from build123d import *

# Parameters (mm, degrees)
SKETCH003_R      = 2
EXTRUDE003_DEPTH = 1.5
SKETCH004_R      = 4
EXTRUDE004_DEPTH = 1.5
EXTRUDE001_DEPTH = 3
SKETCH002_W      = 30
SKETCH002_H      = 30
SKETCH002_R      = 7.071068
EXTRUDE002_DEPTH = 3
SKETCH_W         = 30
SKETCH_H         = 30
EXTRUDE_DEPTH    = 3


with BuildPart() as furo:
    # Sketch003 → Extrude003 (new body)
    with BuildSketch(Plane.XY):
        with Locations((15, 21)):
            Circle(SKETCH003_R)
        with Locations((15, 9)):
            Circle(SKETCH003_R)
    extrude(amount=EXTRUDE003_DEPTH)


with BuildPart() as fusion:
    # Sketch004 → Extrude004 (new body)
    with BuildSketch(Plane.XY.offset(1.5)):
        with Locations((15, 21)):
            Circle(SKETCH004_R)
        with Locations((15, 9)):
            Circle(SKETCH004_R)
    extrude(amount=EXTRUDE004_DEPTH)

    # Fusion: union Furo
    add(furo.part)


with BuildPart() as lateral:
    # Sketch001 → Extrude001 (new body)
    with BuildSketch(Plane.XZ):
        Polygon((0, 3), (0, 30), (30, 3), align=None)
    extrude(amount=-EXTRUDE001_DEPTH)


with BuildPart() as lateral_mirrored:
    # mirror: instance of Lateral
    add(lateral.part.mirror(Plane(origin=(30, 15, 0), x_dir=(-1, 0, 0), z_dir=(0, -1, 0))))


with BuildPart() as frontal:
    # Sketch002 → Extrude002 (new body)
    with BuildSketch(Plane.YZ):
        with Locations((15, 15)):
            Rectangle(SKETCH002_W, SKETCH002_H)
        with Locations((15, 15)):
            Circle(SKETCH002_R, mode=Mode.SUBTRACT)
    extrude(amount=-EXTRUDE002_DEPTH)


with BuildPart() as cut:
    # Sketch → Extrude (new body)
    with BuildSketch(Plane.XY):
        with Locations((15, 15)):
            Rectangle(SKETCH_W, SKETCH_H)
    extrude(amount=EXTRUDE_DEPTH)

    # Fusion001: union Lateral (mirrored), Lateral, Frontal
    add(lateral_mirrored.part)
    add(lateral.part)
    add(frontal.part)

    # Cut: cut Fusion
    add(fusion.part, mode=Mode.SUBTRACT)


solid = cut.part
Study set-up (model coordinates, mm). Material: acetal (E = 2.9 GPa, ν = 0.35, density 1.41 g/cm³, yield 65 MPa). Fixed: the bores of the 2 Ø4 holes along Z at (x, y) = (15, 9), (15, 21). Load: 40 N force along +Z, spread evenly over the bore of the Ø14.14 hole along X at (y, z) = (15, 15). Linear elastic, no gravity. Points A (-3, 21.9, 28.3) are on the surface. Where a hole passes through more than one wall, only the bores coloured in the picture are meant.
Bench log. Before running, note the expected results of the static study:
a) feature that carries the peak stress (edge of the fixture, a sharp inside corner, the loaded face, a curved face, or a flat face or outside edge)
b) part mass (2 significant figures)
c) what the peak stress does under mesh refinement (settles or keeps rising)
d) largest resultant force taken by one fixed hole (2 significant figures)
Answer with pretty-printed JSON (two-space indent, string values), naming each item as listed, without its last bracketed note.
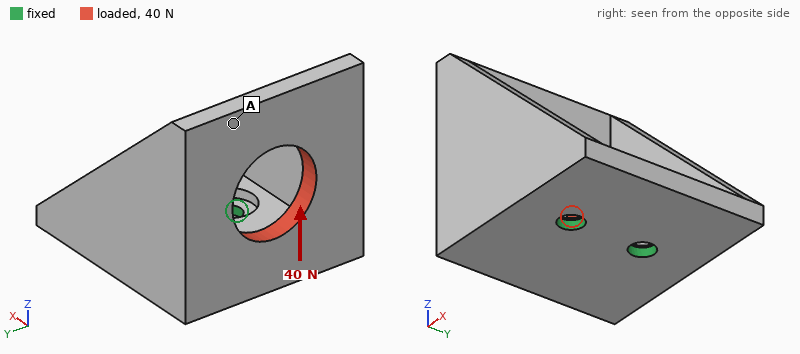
{
  "feature that carries the peak stress": "edge of the fixture",
  "part mass": "10 g",
  "what the peak stress does under mesh refinement": "keeps rising",
  "largest resultant force taken by one fixed hole": "21 N"
}
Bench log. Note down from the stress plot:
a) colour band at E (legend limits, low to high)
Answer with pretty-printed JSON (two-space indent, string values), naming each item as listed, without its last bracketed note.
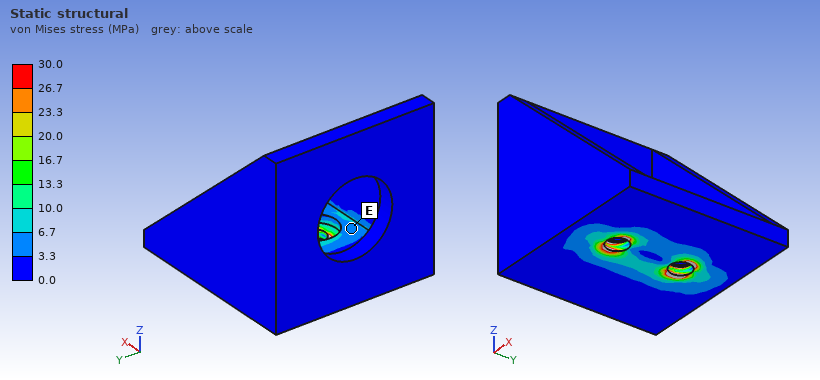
{
  "colour band at E": "3.3 to 6.7 MPa"
}
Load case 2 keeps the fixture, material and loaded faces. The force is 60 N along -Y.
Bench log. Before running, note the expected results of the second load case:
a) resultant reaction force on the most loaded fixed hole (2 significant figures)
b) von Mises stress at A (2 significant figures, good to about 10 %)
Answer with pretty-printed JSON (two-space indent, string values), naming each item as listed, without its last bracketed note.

{
  "resultant reaction force on the most loaded fixed hole": "93 N",
  "von Mises stress at A": "3.3 MPa"
}
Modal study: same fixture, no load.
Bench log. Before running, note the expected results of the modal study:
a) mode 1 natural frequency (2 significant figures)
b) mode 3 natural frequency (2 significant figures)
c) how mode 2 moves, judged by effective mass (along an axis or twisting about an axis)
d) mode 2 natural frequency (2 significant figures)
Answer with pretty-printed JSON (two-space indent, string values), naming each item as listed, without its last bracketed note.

{
  "mode 1 natural frequency": "560 Hz",
  "mode 3 natural frequency": "2200 Hz",
  "how mode 2 moves, judged by effective mass": "along Y",
  "mode 2 natural frequency": "820 Hz"
}
